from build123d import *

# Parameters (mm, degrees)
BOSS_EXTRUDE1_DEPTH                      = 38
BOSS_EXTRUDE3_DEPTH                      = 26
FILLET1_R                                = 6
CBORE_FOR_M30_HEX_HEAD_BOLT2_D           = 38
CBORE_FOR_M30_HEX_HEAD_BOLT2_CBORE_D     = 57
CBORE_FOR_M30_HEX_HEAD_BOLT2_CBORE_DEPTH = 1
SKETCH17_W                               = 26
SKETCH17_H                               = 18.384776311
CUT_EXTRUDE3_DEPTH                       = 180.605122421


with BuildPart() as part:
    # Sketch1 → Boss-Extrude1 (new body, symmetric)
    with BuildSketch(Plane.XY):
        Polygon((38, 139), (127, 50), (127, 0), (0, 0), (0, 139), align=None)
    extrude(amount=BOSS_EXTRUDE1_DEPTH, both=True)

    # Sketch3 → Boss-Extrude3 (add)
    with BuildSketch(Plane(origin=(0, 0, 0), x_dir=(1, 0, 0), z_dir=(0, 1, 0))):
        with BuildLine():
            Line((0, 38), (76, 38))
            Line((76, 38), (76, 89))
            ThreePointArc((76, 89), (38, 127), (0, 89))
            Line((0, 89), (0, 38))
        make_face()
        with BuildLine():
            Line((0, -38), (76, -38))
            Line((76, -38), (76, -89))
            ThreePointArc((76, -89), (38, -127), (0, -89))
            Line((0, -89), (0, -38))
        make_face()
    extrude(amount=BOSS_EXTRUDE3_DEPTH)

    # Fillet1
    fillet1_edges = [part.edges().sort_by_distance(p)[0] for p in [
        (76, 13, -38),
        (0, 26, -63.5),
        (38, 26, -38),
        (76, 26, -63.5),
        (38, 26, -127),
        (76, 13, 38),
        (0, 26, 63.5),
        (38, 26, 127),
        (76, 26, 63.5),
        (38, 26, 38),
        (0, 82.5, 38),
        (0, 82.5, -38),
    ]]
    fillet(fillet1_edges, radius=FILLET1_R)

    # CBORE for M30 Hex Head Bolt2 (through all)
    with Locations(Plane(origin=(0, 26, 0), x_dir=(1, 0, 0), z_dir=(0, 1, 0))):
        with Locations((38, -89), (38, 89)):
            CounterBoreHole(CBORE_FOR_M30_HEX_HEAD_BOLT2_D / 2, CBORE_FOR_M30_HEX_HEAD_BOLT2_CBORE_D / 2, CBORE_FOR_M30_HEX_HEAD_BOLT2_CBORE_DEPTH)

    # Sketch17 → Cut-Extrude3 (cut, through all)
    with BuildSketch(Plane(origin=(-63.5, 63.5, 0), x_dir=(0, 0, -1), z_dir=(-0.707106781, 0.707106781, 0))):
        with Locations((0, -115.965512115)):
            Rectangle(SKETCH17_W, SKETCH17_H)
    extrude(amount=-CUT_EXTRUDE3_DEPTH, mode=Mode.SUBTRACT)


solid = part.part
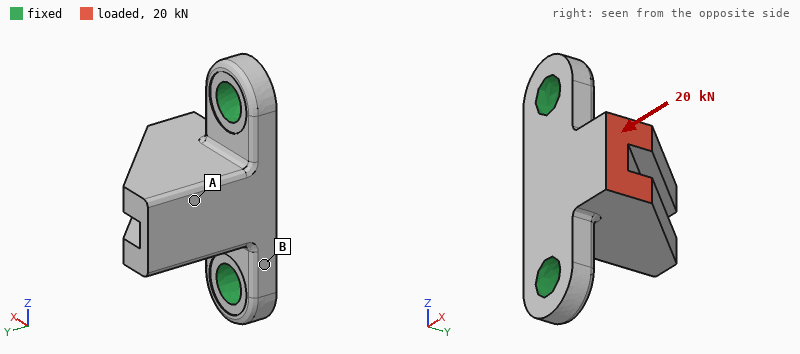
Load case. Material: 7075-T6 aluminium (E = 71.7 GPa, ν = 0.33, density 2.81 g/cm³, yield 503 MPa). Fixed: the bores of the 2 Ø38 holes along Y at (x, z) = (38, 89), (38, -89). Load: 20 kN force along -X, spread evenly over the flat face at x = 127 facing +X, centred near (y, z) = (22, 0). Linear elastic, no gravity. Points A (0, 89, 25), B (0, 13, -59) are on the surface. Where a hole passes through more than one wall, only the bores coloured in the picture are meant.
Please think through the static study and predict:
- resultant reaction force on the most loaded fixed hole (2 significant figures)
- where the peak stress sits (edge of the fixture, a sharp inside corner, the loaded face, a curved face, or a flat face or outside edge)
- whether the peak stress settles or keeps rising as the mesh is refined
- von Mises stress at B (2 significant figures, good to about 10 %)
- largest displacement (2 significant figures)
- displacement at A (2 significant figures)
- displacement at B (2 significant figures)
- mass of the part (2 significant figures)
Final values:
10 kN
edge of the fixture
keeps rising
8.8 MPa
60 µm
43 µm
9.3 µm
3.4 kg
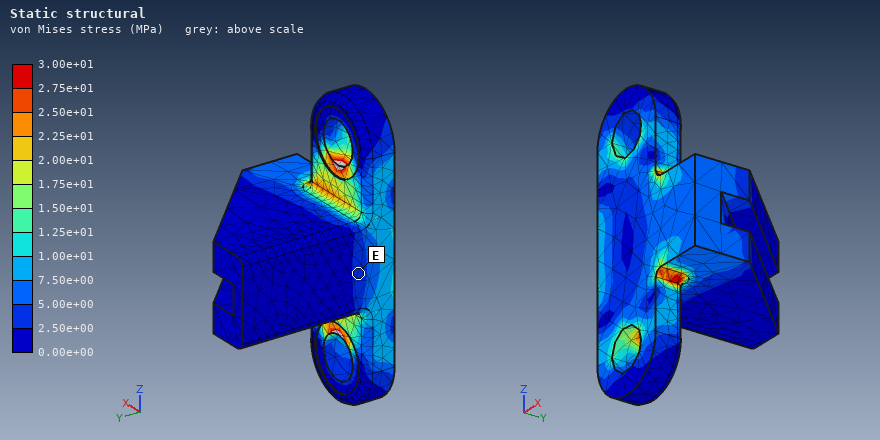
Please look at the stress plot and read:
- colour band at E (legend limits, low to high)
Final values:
2.50e+00 to 5.00e+00 MPa
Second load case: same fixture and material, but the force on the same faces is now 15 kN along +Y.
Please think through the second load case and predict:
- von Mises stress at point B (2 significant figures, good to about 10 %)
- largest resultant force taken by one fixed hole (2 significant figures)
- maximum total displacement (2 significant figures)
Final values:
49 MPa
8.5 kN
0.31 mm
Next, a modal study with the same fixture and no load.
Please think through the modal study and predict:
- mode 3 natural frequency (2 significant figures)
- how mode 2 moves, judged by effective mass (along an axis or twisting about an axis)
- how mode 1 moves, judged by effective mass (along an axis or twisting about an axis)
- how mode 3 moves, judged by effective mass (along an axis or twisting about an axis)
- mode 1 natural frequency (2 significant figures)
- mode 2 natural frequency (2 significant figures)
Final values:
2800 Hz
along Z
along X
along Y
1000 Hz
2400 Hz
